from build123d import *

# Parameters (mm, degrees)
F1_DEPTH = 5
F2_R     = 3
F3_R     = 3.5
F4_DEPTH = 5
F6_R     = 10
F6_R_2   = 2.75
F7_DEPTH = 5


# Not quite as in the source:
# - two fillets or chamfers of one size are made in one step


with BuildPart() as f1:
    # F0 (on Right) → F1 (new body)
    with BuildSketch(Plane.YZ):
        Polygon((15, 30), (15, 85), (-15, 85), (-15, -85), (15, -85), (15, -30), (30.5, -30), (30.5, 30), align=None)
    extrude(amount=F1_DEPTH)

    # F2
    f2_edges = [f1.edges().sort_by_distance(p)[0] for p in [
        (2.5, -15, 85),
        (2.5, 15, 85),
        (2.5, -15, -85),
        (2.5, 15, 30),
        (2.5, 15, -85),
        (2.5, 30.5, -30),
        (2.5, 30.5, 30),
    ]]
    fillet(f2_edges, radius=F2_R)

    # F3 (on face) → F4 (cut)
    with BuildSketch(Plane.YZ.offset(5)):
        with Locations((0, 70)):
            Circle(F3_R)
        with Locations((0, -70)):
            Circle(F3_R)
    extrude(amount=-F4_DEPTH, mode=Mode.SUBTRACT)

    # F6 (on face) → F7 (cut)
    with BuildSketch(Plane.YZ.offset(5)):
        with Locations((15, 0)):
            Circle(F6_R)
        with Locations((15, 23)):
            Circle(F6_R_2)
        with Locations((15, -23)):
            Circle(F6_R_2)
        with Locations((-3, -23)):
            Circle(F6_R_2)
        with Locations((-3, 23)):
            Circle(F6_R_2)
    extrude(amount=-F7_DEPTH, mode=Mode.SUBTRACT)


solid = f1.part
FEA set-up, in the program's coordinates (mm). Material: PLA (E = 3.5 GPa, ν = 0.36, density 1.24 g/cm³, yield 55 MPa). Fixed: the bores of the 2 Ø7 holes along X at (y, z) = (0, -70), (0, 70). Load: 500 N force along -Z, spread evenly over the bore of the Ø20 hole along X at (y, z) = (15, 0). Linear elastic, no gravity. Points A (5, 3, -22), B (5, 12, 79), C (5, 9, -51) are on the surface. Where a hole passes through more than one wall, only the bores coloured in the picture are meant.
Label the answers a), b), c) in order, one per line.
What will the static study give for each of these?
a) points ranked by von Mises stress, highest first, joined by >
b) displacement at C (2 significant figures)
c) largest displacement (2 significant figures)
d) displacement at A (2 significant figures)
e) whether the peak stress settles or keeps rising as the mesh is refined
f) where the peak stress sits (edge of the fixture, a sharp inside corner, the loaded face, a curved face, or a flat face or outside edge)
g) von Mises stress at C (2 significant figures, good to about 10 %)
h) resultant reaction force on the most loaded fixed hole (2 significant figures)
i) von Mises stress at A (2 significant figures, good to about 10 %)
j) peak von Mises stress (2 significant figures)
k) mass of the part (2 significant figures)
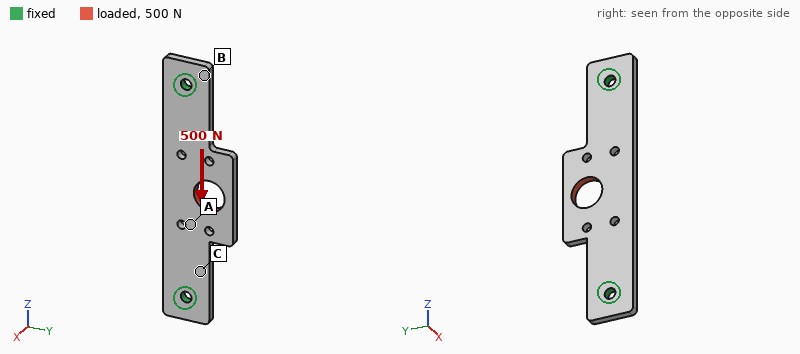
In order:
a) C > A > B
b) 14 µm
c) 74 µm
d) 30 µm
e) settles
f) a curved face
g) 2.4 MPa
h) 260 N
i) 1.5 MPa
j) 12 MPa
k) 34 g
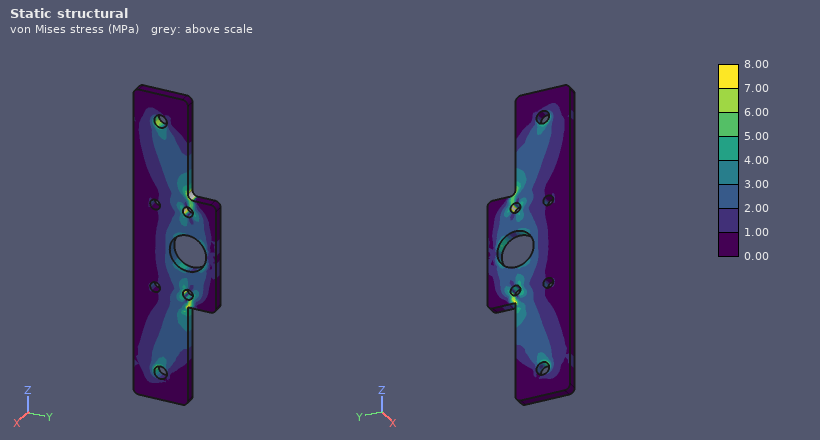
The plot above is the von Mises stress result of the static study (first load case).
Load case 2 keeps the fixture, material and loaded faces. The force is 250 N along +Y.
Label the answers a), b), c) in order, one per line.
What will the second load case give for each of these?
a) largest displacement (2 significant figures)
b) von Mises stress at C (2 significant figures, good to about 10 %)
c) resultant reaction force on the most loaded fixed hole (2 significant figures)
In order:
a) 0.17 mm
b) 1.4 MPa
c) 130 N
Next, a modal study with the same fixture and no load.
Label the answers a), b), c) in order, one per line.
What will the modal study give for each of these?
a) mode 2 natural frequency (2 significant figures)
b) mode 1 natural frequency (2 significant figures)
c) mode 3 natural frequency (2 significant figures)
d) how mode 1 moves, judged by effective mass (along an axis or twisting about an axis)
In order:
a) 740 Hz
b) 390 Hz
c) 1100 Hz
d) along X
